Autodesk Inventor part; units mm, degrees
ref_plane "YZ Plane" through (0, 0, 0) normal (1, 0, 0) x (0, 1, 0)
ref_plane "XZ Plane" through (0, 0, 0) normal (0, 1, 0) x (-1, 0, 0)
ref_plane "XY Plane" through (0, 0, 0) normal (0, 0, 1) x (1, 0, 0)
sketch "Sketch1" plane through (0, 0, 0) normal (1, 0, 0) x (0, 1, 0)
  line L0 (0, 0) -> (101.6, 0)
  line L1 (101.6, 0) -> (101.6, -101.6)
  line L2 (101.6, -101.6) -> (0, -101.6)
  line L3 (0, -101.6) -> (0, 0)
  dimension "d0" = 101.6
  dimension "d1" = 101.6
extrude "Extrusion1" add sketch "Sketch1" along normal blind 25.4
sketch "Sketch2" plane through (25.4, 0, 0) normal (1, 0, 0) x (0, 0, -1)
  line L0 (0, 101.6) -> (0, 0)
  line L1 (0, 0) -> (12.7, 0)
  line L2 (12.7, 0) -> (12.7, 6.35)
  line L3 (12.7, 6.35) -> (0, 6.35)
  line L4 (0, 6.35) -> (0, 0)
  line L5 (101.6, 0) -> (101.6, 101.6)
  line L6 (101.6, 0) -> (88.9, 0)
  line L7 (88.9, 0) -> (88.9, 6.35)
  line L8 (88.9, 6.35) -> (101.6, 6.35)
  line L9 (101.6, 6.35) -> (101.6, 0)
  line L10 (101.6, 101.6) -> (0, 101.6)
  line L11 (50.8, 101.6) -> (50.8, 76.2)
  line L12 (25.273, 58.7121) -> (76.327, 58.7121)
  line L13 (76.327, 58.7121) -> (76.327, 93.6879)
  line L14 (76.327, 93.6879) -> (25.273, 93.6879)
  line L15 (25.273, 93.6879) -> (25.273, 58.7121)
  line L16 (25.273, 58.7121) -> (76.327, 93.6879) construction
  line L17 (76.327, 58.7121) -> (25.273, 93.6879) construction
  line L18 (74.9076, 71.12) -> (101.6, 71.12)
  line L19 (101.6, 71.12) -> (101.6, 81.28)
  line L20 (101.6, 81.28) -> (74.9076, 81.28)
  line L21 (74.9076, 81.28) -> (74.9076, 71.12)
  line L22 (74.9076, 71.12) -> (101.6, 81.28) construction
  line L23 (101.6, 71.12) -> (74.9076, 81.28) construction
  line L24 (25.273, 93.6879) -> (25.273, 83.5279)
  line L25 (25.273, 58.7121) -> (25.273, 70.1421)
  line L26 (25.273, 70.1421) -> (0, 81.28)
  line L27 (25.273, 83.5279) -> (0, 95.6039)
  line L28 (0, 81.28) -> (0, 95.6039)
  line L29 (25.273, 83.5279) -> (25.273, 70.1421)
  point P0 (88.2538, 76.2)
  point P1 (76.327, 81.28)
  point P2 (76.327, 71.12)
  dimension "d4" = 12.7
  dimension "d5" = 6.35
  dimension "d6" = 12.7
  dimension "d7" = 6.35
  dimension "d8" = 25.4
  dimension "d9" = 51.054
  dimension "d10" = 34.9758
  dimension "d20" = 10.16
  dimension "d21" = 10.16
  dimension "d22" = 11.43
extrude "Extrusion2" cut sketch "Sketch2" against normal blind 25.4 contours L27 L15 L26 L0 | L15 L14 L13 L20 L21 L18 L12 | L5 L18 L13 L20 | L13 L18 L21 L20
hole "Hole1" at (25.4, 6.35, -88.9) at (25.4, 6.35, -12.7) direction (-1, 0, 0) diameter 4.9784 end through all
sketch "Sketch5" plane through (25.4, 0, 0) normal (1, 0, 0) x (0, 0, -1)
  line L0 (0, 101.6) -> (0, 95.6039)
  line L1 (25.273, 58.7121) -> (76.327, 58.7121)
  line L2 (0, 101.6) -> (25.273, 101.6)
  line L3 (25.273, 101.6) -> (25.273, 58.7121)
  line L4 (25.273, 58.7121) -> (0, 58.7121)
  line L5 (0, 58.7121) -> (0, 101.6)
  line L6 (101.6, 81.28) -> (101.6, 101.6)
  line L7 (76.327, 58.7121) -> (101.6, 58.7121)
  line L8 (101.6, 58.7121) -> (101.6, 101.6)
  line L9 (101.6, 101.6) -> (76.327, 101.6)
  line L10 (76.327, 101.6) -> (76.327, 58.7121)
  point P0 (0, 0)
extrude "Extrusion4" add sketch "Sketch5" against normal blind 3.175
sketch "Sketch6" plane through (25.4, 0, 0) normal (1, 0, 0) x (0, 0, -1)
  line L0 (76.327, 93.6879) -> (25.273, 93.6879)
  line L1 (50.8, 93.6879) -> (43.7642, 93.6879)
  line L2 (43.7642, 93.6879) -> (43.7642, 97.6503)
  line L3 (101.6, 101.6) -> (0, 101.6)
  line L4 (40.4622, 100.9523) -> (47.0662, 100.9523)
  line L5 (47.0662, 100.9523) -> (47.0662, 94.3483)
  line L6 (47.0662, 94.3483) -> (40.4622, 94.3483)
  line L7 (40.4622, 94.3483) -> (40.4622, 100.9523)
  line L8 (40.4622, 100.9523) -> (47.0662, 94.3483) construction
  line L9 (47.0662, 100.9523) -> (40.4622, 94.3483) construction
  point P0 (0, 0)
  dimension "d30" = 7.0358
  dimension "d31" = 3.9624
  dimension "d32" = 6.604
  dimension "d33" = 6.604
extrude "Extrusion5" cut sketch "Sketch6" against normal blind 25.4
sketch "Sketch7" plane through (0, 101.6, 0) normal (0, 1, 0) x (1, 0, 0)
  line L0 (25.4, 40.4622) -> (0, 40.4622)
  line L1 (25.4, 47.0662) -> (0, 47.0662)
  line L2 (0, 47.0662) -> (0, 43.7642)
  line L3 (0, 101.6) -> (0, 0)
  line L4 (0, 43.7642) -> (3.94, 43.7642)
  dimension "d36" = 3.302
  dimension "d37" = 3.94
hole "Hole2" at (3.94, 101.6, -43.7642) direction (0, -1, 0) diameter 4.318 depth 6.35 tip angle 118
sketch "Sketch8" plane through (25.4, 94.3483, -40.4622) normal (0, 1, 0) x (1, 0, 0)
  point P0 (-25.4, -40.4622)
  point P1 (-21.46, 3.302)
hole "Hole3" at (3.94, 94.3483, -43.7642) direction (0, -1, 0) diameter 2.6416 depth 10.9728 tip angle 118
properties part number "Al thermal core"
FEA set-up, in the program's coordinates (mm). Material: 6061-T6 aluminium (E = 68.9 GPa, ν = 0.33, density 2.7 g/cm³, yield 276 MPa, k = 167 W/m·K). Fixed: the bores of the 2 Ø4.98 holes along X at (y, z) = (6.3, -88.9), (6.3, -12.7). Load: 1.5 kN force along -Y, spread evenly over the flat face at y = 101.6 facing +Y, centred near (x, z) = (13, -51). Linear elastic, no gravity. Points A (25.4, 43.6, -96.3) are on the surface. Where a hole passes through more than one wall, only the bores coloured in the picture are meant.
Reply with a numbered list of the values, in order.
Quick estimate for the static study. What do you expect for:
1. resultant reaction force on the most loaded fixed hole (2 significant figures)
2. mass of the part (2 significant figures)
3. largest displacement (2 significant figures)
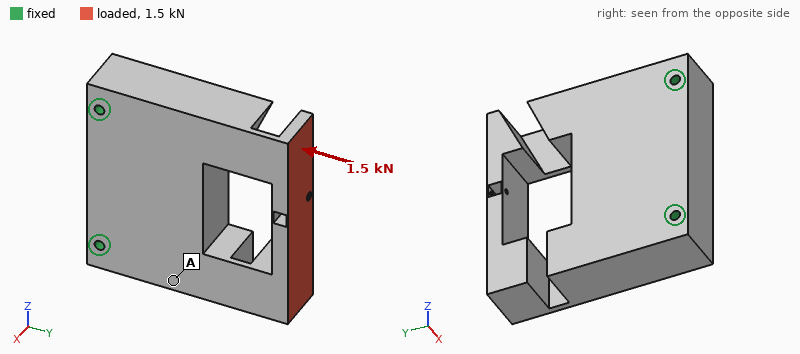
1. 750 N
2. 540 g
3. 0.72 mm
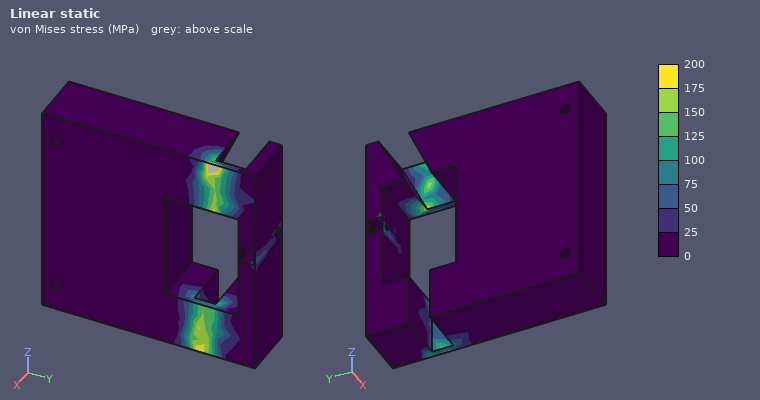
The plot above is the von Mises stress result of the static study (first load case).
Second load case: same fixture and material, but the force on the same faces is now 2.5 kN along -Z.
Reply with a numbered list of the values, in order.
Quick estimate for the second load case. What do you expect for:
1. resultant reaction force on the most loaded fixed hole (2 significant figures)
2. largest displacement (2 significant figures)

1. 3.3 kN
2. 0.19 mm
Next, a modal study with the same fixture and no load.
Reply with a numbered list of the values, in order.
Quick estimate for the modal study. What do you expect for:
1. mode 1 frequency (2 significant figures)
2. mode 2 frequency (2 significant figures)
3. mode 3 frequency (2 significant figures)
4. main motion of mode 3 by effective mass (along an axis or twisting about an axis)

1. 720 Hz
2. 2100 Hz
3. 2500 Hz
4. along X
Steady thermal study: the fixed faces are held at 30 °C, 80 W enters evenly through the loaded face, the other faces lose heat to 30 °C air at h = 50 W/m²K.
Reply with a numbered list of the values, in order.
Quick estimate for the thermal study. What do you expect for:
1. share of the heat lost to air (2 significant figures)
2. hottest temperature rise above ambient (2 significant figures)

1. 36 %
2. 68 K
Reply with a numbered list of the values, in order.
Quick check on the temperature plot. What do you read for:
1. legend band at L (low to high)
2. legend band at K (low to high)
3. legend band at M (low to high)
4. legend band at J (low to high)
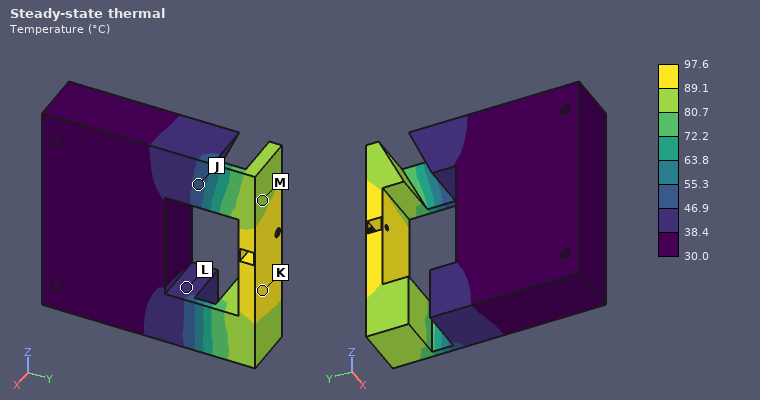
1. 38.4 to 46.9 °C
2. 89.1 to 97.6 °C
3. 80.7 to 89.1 °C
4. 46.9 to 55.3 °C
